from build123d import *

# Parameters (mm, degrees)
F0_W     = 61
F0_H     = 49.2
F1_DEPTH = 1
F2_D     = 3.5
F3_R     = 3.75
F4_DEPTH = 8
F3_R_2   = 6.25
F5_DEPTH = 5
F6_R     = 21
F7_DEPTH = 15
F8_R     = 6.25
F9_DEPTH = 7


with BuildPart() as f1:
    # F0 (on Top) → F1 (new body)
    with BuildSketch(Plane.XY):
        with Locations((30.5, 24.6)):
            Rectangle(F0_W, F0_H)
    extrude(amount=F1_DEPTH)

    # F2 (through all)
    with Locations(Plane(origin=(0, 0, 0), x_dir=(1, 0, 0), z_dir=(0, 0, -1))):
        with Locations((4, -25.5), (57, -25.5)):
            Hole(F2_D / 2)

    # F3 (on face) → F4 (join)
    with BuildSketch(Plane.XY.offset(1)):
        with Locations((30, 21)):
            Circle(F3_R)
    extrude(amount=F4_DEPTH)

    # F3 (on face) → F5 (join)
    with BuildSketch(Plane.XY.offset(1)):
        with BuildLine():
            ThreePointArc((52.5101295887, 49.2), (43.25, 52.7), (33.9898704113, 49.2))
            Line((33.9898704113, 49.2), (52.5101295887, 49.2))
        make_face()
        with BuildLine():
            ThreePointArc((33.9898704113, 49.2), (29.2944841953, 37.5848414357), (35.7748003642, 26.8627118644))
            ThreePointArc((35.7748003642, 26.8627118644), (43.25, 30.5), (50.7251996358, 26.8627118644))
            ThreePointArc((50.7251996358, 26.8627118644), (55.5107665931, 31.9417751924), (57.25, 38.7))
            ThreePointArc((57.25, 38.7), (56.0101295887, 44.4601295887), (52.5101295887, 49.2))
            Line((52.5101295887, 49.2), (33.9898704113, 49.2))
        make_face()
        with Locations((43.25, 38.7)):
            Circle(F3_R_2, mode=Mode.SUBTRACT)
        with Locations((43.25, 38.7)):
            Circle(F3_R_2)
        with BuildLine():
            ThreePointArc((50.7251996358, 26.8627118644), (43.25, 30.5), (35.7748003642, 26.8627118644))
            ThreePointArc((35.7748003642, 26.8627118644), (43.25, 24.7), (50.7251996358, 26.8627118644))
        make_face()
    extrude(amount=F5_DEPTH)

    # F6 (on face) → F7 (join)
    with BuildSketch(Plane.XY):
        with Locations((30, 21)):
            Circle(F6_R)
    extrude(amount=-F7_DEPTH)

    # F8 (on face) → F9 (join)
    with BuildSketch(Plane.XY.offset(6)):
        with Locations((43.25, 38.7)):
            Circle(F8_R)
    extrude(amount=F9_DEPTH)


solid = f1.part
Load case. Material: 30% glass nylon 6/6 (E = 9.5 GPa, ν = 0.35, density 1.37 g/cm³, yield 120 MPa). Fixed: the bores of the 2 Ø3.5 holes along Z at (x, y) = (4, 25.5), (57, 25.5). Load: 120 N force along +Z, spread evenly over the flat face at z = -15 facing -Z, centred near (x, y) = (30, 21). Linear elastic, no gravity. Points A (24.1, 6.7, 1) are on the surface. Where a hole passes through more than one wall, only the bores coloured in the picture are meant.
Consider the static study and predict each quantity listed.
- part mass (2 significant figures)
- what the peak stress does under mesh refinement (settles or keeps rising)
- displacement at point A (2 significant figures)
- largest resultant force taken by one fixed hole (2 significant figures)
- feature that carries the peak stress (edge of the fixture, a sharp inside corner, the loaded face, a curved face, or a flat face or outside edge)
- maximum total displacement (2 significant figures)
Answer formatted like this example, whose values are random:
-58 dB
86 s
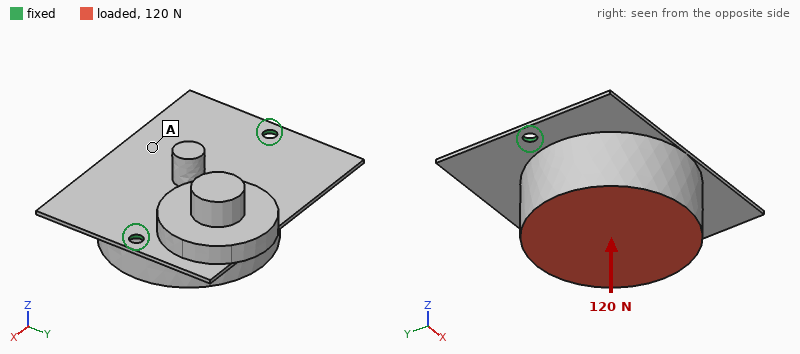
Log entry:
38 g
keeps rising
0.62 mm
67 N
edge of the fixture
0.95 mm
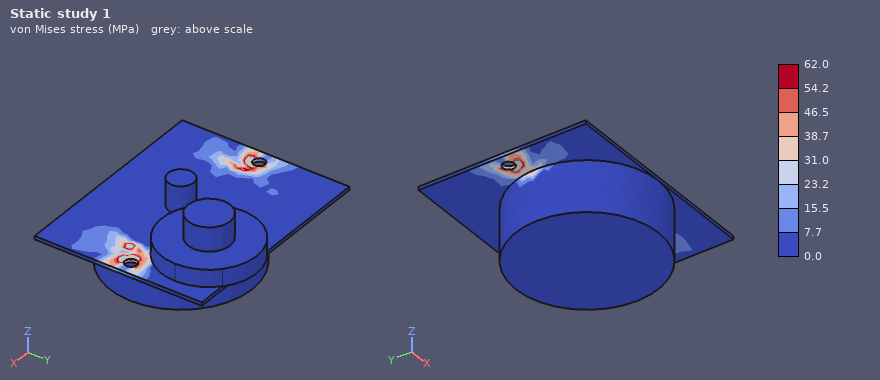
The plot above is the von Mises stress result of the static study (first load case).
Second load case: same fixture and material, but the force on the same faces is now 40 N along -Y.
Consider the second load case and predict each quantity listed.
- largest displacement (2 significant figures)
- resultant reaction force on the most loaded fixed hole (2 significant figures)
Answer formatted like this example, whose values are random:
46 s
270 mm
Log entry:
0.97 mm
23 N
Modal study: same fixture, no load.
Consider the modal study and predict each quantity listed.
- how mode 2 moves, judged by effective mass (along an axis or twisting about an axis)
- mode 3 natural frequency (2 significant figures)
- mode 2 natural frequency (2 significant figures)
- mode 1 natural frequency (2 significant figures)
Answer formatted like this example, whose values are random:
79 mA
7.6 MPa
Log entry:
along Z
1800 Hz
1100 Hz
240 Hz
